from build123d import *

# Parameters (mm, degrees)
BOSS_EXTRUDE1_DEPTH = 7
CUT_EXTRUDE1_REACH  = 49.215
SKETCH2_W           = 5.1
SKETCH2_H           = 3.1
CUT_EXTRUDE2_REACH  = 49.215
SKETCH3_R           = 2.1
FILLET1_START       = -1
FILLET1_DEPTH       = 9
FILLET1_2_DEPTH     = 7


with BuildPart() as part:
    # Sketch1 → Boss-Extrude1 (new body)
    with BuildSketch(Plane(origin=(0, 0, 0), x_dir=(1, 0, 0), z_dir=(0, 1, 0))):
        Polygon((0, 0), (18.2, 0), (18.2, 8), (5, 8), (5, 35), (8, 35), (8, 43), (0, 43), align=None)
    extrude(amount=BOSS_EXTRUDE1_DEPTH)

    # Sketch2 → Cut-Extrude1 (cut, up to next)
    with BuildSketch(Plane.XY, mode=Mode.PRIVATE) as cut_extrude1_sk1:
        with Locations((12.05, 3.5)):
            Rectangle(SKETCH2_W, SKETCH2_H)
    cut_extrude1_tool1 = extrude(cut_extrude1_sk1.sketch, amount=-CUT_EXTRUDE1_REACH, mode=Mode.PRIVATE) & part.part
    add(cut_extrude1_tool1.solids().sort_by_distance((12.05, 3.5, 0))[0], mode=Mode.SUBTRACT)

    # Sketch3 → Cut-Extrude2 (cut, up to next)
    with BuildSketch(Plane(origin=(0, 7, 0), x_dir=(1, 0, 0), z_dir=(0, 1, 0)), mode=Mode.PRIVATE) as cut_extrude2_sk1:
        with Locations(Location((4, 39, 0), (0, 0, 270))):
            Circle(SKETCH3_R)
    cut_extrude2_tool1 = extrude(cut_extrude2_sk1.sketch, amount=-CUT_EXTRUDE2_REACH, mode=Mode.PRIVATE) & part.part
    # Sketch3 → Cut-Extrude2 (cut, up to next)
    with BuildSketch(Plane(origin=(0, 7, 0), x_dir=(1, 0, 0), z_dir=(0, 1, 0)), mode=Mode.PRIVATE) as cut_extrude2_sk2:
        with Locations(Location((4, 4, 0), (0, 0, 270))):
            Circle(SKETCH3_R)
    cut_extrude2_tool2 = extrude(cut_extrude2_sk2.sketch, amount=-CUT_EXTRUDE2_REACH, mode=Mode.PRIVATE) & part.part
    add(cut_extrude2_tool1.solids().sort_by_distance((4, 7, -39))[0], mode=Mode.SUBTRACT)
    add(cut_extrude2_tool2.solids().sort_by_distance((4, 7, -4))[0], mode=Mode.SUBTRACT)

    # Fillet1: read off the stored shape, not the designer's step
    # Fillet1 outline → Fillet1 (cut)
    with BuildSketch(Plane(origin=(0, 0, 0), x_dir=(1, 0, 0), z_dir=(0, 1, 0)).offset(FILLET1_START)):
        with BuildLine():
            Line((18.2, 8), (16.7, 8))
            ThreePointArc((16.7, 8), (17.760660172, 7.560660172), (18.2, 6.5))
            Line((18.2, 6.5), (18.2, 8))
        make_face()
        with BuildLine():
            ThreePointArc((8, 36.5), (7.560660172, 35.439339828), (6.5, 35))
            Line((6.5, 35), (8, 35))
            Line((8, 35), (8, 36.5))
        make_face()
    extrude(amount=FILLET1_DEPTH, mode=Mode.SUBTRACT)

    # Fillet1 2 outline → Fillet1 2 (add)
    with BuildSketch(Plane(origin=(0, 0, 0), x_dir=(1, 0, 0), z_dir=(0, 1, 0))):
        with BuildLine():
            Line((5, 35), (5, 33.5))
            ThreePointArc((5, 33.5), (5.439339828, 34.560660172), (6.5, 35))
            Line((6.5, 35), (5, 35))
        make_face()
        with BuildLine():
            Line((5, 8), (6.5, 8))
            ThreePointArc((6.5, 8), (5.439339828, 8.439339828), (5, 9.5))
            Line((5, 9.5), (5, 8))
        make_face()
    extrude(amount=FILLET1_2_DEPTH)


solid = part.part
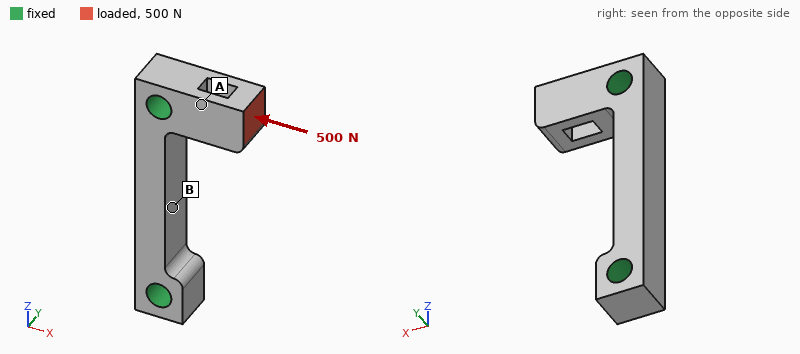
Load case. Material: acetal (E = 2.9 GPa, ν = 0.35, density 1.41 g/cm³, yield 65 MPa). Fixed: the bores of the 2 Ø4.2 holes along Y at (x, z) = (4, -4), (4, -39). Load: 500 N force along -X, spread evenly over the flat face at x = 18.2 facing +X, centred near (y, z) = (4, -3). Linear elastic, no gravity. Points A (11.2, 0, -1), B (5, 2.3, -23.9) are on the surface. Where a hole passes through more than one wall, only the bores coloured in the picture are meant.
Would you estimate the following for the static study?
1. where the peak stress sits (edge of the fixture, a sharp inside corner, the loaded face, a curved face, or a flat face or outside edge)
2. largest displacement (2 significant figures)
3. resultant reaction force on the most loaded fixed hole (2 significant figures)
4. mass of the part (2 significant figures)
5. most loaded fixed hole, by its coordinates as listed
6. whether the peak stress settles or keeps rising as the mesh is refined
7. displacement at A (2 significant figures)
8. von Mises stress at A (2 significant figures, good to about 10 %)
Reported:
a sharp inside corner
0.12 mm
500 N
2.9 g
(4, -4)
keeps rising
0.050 mm
17 MPa
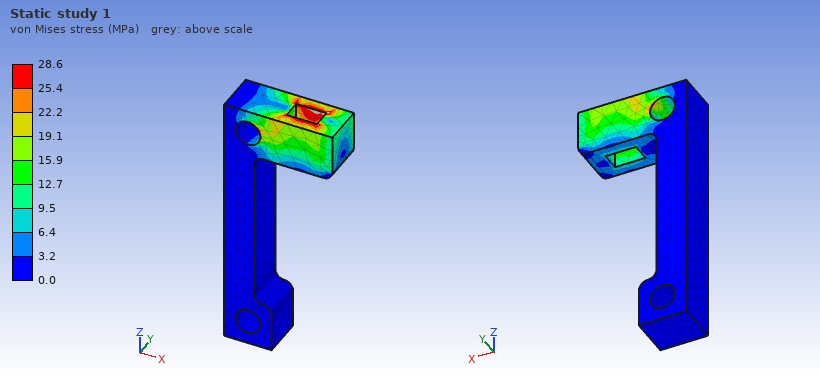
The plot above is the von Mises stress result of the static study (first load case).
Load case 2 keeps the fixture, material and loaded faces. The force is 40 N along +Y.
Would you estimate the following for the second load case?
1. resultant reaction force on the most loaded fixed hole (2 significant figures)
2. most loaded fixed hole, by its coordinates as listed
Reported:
40 N
(4, -4)
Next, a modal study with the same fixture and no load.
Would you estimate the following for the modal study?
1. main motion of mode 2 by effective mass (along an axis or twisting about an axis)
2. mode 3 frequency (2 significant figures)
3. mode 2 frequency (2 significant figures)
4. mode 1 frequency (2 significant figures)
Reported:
along X
7600 Hz
6600 Hz
6200 Hz
